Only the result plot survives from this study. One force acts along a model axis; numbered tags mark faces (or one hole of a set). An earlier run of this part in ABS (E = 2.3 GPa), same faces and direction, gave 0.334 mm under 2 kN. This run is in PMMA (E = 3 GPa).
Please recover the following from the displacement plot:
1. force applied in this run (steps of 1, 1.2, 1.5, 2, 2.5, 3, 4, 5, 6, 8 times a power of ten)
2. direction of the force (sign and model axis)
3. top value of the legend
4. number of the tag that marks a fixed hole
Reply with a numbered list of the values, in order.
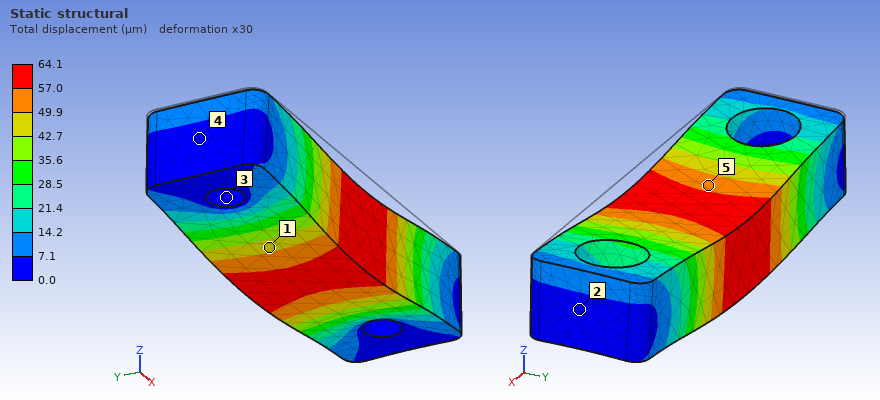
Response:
1. 500 N
2. -Z
3. 64.1 µm
4. 3
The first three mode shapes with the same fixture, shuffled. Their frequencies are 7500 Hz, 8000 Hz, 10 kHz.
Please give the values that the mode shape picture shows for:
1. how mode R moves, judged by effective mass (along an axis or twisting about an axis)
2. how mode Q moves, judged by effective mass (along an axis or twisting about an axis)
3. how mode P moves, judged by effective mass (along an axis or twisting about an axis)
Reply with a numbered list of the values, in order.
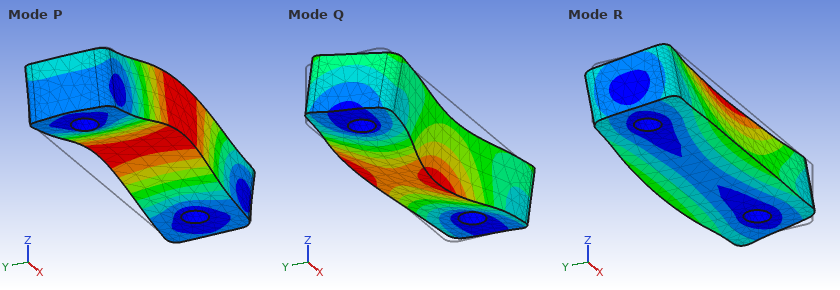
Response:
1. along Y
2. along Y
3. along Z
